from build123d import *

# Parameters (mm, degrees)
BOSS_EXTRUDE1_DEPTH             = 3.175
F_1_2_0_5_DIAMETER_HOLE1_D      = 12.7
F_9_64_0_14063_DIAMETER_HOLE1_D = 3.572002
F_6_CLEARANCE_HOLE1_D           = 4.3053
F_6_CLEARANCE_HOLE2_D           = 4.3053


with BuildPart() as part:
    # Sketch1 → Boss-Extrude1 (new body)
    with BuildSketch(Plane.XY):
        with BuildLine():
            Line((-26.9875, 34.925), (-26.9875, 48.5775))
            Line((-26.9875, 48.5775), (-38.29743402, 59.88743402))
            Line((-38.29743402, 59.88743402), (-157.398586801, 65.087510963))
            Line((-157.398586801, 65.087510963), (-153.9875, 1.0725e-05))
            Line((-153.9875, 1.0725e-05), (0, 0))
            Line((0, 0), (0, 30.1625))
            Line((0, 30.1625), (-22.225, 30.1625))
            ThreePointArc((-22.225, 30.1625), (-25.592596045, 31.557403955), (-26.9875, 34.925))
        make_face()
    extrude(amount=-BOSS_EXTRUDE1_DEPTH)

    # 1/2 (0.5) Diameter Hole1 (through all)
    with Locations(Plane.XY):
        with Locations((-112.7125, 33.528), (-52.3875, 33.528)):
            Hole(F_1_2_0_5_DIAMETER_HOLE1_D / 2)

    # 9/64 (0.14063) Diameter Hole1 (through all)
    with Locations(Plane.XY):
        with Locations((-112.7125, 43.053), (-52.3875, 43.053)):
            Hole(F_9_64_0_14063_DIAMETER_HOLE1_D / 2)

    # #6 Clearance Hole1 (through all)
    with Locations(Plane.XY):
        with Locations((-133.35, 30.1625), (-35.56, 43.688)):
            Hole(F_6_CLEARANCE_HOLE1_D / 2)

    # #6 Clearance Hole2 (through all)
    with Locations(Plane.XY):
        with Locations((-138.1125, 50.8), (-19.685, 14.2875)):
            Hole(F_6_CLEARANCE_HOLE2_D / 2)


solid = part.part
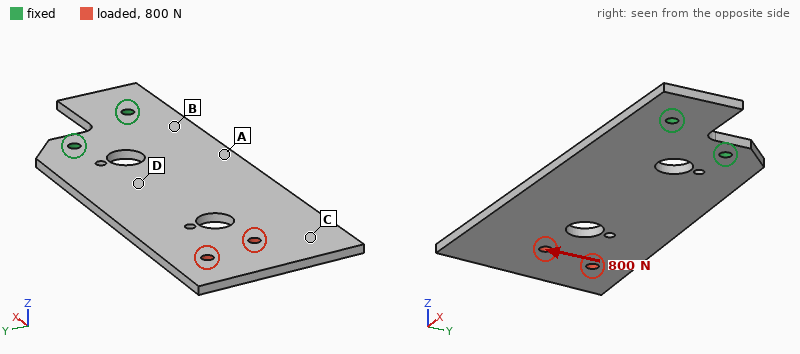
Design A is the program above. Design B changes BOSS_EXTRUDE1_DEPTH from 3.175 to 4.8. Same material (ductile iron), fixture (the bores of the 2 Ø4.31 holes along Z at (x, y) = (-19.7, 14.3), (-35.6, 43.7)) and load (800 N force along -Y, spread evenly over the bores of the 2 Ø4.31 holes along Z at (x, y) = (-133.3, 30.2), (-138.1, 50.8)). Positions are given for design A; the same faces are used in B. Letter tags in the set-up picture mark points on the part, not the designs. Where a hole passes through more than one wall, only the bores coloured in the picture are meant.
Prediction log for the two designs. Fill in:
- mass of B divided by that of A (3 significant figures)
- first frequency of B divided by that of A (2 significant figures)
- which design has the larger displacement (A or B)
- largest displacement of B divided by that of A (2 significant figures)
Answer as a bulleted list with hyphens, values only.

- 1.51
- 1.5
- A
- 0.66
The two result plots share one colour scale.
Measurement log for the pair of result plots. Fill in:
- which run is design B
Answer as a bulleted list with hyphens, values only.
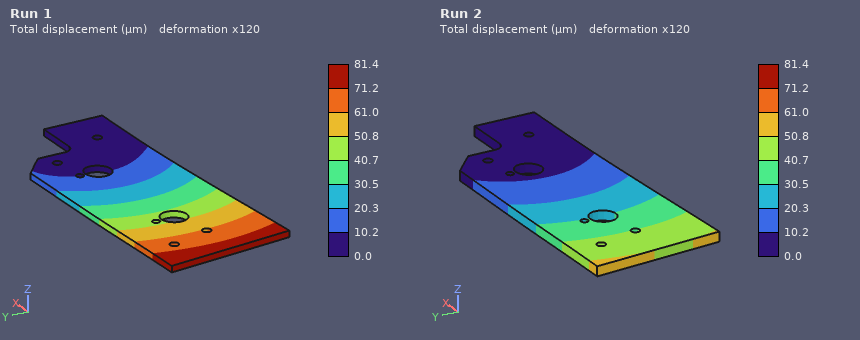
- Run 2
